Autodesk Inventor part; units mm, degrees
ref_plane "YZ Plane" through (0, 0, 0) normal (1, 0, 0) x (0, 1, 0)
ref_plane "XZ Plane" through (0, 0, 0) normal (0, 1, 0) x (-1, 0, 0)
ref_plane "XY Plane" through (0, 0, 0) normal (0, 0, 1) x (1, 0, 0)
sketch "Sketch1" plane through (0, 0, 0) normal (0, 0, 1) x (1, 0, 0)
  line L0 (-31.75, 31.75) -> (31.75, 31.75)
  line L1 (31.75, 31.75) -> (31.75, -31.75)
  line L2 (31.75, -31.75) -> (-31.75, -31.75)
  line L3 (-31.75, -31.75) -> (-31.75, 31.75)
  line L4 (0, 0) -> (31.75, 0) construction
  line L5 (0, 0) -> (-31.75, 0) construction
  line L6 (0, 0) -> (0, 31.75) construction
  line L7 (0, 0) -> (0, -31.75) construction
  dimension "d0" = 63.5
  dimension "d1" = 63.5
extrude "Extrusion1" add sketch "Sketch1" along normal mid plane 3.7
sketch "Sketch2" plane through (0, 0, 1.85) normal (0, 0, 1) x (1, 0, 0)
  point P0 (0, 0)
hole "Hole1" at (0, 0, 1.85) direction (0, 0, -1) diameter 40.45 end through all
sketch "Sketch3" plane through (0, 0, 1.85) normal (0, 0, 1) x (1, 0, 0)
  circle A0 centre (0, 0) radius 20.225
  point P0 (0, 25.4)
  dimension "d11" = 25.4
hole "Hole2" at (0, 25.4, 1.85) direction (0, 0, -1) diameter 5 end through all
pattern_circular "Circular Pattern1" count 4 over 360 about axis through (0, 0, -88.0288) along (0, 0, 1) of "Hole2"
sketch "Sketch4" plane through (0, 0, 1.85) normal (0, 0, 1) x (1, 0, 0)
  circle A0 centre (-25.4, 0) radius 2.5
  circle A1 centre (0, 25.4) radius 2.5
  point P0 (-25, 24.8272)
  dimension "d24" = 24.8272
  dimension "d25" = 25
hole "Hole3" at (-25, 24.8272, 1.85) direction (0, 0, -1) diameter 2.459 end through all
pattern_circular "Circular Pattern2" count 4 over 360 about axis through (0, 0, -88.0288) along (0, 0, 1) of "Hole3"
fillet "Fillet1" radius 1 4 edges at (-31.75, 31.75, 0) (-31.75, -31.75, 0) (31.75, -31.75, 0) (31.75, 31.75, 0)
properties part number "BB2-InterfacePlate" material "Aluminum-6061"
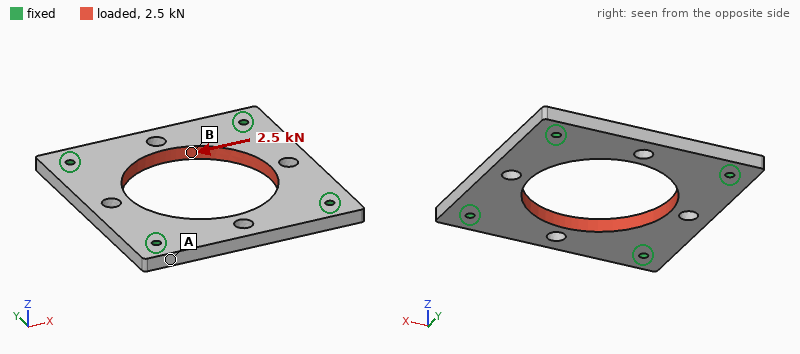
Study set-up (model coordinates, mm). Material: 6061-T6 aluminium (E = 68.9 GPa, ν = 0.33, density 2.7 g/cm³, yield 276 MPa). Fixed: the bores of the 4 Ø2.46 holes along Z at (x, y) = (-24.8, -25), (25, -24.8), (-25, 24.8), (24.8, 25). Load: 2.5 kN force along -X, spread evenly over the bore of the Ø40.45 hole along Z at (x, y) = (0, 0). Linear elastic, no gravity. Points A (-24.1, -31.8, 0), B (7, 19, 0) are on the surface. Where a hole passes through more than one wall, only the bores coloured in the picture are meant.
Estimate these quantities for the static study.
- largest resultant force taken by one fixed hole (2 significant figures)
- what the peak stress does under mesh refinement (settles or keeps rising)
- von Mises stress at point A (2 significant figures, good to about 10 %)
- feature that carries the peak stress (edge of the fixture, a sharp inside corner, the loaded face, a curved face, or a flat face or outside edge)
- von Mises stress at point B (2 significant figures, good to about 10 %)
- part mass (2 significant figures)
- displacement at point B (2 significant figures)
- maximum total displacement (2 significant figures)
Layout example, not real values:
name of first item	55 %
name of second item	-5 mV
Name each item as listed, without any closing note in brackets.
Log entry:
largest resultant force taken by one fixed hole	640 N
what the peak stress does under mesh refinement	keeps rising
von Mises stress at point A	6.9 MPa
feature that carries the peak stress	edge of the fixture
von Mises stress at point B	15 MPa
part mass	26 g
displacement at point B	4.4 µm
maximum total displacement	12 µm
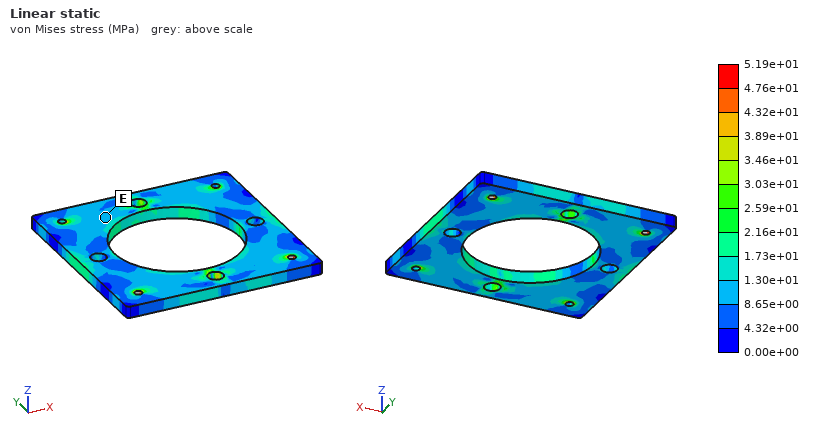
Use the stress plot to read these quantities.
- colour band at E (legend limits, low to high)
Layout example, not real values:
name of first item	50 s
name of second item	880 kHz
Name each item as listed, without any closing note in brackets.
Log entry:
colour band at E	8.65e+00 to 1.30e+01 MPa
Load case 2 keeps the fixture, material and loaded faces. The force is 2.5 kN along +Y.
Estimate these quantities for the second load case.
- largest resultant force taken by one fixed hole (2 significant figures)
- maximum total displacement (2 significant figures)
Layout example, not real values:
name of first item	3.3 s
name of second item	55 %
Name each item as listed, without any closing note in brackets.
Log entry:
largest resultant force taken by one fixed hole	640 N
maximum total displacement	12 µm
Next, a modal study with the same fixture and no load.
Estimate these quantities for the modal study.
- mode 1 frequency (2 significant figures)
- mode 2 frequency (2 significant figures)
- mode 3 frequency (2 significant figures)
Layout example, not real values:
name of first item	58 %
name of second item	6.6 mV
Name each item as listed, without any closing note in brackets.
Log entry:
mode 1 frequency	7300 Hz
mode 2 frequency	7300 Hz
mode 3 frequency	7700 Hz
